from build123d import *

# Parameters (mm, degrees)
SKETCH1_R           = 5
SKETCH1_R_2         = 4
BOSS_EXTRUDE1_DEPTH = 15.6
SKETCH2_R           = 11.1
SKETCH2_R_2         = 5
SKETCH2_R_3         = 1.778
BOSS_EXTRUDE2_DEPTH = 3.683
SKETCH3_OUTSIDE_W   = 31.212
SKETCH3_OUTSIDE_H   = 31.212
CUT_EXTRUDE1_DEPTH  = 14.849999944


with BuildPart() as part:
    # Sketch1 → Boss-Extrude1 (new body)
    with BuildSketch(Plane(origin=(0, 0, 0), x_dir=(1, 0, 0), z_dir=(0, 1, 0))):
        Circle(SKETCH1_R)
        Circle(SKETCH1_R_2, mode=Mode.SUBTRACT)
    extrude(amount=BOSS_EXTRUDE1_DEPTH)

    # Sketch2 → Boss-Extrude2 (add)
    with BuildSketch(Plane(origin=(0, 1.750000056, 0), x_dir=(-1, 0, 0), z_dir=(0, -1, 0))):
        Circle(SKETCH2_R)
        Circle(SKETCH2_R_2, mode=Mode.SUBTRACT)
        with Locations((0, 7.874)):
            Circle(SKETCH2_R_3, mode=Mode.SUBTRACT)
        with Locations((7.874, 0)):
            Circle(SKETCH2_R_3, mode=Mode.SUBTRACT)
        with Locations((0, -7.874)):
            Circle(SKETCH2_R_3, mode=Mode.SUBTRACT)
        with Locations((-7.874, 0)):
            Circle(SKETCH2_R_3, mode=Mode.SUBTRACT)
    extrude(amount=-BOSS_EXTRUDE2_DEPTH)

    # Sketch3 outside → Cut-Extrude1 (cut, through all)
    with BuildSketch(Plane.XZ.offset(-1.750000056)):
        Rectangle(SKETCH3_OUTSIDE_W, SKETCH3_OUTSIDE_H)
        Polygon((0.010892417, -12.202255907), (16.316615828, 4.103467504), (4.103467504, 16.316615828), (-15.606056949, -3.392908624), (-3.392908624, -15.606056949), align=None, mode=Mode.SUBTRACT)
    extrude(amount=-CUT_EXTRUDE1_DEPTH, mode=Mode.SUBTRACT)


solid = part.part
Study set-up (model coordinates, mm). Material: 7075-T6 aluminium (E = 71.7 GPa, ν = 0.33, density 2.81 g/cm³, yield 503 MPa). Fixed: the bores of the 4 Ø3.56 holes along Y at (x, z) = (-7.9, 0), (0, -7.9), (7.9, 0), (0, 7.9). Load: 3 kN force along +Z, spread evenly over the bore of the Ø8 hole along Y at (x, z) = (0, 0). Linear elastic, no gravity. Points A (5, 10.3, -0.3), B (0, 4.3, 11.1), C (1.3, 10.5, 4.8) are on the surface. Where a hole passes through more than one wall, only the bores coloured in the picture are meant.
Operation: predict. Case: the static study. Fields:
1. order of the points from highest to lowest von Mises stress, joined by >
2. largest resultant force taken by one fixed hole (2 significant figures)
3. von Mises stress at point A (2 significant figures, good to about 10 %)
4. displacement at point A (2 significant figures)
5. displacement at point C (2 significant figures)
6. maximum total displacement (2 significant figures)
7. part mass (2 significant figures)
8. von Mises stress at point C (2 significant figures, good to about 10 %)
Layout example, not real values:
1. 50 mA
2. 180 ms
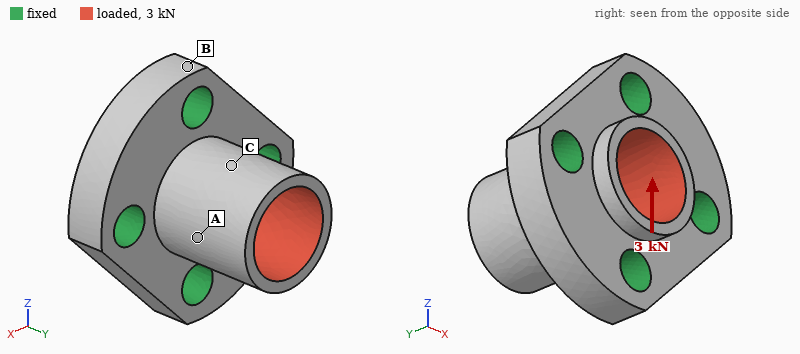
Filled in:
1. A > C > B
2. 1.3 kN
3. 120 MPa
4. 29 µm
5. 35 µm
6. 55 µm
7. 3.5 g
8. 57 MPa
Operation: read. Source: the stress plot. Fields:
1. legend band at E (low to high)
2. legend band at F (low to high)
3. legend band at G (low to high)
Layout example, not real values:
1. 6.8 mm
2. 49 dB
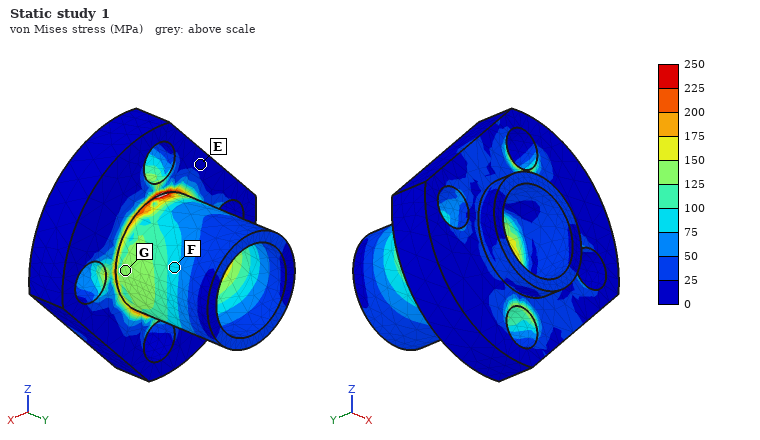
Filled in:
1. 0 to 25 MPa
2. 75 to 100 MPa
3. 125 to 150 MPa
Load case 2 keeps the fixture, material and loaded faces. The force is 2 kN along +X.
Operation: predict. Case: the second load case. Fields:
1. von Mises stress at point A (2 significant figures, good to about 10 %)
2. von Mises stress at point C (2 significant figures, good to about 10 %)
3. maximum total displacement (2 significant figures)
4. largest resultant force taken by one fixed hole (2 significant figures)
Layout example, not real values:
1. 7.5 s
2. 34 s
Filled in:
1. 35 MPa
2. 72 MPa
3. 36 µm
4. 840 N
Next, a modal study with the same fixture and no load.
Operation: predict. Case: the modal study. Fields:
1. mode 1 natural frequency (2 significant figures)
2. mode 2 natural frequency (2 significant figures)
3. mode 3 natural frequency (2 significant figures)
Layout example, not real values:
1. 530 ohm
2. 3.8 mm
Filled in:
1. 39 kHz
2. 39 kHz
3. 39 kHz
